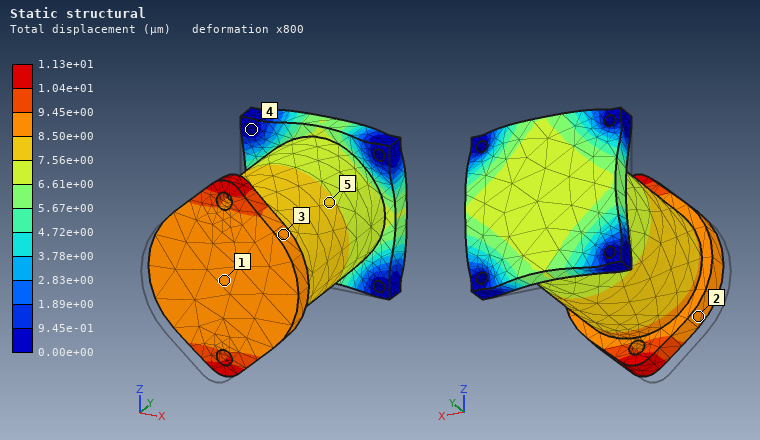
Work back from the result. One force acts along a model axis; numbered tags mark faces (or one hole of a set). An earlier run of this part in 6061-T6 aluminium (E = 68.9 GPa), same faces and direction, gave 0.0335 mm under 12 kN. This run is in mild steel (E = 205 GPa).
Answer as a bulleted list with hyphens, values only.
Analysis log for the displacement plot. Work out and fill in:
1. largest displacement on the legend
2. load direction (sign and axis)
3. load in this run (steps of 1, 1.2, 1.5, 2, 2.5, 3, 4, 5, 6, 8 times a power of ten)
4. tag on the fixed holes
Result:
- 1.13e+01 µm
- +Y
- 12 kN
- 4
